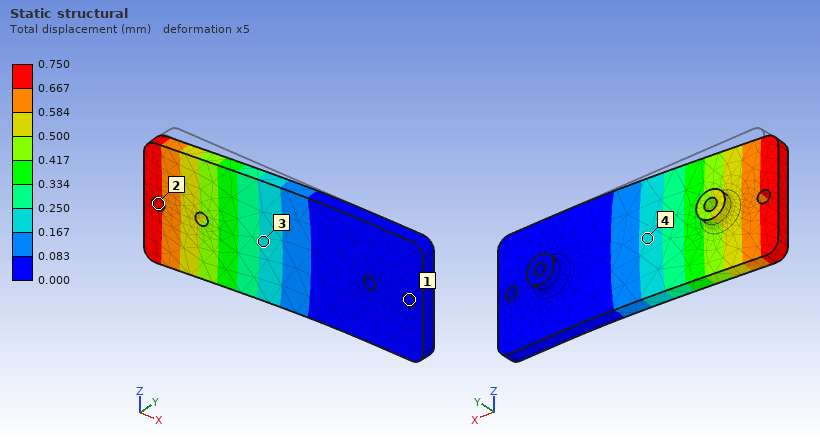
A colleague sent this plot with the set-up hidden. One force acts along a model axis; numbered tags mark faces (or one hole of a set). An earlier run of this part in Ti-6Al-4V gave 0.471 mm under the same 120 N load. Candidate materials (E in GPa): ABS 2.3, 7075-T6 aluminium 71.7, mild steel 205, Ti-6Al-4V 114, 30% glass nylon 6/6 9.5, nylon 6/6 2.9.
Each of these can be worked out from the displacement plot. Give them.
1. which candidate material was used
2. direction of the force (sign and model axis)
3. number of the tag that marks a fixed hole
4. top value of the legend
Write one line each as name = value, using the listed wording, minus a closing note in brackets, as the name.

which candidate material was used = 7075-T6 aluminium
direction of the force = -Y
number of the tag that marks a fixed hole = 1
top value of the legend = 0.750 mm
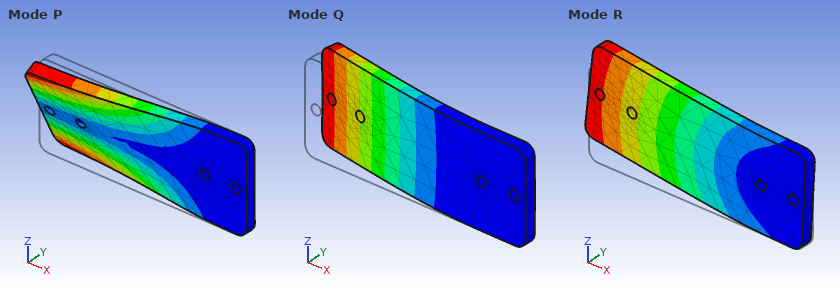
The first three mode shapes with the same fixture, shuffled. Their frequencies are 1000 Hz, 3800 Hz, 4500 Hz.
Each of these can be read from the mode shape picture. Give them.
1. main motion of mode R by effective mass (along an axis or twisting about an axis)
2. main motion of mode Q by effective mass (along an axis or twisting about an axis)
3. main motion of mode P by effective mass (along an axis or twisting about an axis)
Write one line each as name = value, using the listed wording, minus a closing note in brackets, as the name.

main motion of mode R by effective mass = along Z
main motion of mode Q by effective mass = along Y
main motion of mode P by effective mass = twisting about X
